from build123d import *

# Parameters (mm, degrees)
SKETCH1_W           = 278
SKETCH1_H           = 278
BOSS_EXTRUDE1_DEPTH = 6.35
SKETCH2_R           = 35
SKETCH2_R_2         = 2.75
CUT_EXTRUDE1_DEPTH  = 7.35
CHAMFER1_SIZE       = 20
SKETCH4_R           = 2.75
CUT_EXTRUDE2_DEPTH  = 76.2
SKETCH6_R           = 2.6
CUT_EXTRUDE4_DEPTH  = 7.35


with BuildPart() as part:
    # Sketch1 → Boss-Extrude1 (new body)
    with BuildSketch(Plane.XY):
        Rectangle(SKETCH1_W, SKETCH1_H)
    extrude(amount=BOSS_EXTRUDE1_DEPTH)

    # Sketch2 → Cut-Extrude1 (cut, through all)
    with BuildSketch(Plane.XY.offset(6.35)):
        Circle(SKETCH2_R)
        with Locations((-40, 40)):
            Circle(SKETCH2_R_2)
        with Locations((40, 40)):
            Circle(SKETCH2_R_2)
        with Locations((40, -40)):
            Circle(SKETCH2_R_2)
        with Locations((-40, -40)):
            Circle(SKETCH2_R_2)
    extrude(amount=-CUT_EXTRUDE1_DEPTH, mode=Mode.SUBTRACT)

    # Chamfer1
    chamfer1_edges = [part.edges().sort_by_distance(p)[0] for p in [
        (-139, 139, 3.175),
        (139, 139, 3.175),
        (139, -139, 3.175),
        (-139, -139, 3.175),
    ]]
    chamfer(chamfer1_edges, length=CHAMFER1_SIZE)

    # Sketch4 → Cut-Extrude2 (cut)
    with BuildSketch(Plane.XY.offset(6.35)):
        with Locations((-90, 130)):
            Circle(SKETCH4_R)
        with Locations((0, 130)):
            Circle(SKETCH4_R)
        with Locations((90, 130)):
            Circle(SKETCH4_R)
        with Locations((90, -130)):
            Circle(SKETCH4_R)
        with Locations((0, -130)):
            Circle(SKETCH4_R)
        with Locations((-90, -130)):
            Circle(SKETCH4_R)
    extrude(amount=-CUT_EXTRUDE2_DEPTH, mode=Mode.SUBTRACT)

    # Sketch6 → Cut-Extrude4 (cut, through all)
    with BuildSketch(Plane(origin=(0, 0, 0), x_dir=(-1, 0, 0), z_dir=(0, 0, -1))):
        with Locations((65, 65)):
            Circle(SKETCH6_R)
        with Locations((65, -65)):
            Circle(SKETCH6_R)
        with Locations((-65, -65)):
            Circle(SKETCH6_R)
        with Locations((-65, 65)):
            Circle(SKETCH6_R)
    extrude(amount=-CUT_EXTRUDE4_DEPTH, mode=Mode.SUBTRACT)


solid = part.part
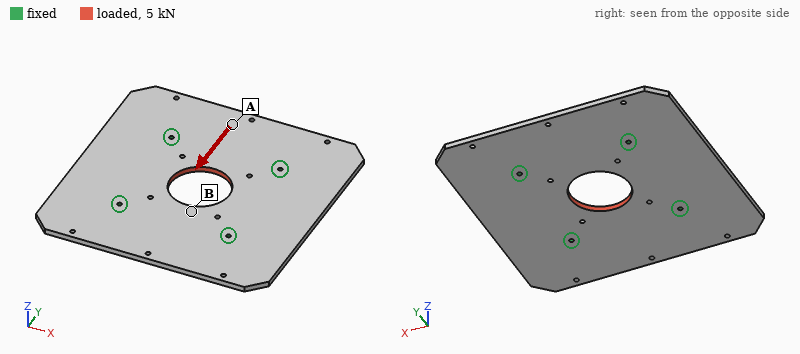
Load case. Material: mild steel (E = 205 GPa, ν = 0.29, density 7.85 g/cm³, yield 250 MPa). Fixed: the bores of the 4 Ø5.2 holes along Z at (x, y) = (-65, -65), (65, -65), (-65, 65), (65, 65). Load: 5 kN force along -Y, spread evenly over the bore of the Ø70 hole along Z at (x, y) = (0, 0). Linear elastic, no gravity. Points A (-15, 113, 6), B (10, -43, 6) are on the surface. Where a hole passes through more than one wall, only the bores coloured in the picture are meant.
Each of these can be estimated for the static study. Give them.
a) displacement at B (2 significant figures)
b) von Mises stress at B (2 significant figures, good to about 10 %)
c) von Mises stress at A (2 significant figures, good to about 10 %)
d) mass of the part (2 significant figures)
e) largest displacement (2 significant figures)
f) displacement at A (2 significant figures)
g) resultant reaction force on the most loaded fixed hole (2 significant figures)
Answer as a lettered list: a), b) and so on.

a) 1.7 µm
b) 3.1 MPa
c) 1.3 MPa
d) 3.6 kg
e) 1.9 µm
f) 1.1 µm
g) 1.3 kN
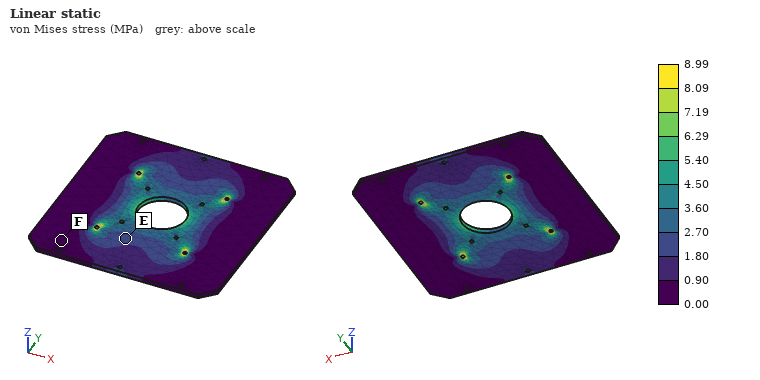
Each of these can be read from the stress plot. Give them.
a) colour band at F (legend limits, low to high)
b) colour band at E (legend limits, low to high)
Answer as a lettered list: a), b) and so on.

a) 0.00 to 0.90 MPa
b) 1.80 to 2.70 MPa
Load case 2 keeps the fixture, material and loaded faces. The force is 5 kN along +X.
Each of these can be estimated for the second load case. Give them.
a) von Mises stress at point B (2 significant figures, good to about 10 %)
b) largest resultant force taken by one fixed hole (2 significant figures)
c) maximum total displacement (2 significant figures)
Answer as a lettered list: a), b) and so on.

a) 4.4 MPa
b) 1.3 kN
c) 1.9 µm
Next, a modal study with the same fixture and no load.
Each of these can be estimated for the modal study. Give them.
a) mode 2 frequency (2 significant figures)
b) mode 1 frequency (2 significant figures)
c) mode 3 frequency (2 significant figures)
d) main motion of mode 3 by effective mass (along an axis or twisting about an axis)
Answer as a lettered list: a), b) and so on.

a) 670 Hz
b) 660 Hz
c) 710 Hz
d) twisting about Y
